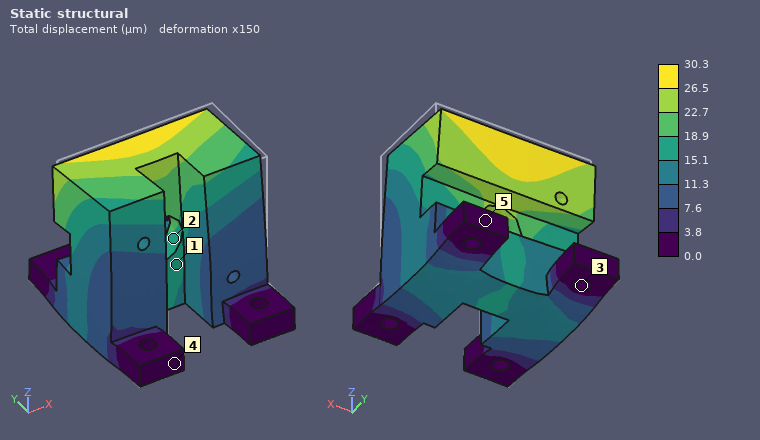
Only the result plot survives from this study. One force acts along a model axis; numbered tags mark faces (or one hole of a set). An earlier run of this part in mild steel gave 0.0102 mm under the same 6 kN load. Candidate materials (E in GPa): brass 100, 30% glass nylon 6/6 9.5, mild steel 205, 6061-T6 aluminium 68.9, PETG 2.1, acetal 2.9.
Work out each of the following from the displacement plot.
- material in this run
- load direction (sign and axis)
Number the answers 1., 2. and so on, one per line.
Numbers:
1. 6061-T6 aluminium
2. -Z
